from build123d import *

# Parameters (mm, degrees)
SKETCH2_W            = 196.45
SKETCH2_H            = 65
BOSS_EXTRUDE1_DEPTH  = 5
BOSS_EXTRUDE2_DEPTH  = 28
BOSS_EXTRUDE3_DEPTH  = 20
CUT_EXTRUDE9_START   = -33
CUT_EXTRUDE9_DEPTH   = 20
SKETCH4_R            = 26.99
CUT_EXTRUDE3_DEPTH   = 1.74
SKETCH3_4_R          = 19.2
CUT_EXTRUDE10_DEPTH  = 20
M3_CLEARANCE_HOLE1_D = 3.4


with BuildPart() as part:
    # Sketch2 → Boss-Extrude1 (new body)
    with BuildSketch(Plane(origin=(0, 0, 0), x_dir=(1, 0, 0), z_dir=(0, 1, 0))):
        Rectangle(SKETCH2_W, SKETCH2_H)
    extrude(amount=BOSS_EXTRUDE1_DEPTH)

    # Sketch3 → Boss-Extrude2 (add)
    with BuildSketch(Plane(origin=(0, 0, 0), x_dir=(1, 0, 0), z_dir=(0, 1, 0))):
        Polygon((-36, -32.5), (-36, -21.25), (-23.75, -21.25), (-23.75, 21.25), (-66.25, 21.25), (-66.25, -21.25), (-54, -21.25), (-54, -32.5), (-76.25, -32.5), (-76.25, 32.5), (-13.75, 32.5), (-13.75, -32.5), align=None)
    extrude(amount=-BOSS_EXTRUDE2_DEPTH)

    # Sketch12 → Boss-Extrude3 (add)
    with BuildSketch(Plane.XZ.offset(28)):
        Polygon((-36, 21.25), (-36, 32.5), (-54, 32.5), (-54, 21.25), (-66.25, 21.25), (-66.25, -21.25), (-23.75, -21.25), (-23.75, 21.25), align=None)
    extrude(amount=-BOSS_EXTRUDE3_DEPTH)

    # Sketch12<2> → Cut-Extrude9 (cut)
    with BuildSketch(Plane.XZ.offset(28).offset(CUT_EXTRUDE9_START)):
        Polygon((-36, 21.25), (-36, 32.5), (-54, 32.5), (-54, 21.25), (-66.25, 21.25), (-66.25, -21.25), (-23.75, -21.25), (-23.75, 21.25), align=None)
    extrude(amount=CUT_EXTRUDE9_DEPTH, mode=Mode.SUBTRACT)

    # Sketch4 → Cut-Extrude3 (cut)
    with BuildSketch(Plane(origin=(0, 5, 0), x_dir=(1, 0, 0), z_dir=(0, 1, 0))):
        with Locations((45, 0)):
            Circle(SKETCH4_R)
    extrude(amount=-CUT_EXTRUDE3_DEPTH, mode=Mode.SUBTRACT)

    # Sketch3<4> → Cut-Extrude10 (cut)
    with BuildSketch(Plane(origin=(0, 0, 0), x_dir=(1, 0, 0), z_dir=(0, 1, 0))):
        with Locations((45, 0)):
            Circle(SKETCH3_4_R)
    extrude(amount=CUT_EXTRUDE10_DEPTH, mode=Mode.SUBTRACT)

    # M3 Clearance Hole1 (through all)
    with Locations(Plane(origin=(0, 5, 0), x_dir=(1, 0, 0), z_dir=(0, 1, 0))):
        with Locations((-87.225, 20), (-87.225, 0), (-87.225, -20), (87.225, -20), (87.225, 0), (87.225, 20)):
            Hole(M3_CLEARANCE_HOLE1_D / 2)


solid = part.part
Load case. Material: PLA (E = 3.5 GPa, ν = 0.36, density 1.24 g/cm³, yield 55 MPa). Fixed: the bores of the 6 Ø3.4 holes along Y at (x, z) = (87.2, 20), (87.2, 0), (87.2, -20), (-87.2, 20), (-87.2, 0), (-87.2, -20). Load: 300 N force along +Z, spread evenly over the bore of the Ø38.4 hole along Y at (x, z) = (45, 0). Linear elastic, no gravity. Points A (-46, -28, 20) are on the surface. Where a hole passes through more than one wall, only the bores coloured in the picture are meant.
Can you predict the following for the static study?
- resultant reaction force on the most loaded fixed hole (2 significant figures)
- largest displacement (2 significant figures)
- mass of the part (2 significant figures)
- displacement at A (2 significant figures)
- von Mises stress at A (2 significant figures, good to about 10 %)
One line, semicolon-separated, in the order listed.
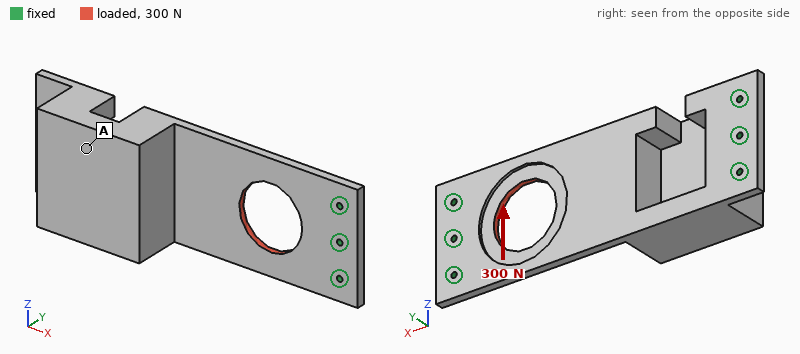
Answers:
120 N; 0.12 mm; 160 g; 0.034 mm; 0.59 MPa
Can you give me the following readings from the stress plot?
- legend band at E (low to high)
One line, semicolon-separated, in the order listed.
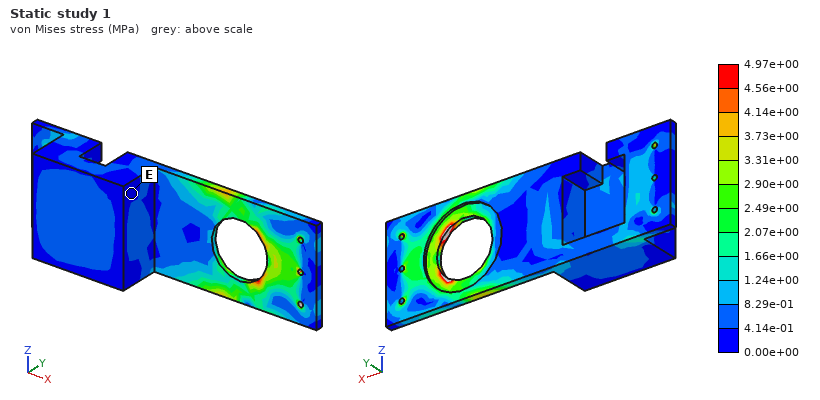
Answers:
0.00e+00 to 4.14e-01 MPa
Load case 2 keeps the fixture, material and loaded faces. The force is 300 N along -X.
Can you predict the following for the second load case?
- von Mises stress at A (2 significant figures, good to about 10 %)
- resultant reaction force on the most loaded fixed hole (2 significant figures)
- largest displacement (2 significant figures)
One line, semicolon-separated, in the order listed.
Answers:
0.30 MPa; 98 N; 45 µm
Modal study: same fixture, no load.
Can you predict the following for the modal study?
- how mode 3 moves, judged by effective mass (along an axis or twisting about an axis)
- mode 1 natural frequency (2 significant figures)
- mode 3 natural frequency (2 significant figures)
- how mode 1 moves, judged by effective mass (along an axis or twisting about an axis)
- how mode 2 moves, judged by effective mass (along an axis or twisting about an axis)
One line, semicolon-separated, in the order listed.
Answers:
along Z; 190 Hz; 840 Hz; along Y; along Z
